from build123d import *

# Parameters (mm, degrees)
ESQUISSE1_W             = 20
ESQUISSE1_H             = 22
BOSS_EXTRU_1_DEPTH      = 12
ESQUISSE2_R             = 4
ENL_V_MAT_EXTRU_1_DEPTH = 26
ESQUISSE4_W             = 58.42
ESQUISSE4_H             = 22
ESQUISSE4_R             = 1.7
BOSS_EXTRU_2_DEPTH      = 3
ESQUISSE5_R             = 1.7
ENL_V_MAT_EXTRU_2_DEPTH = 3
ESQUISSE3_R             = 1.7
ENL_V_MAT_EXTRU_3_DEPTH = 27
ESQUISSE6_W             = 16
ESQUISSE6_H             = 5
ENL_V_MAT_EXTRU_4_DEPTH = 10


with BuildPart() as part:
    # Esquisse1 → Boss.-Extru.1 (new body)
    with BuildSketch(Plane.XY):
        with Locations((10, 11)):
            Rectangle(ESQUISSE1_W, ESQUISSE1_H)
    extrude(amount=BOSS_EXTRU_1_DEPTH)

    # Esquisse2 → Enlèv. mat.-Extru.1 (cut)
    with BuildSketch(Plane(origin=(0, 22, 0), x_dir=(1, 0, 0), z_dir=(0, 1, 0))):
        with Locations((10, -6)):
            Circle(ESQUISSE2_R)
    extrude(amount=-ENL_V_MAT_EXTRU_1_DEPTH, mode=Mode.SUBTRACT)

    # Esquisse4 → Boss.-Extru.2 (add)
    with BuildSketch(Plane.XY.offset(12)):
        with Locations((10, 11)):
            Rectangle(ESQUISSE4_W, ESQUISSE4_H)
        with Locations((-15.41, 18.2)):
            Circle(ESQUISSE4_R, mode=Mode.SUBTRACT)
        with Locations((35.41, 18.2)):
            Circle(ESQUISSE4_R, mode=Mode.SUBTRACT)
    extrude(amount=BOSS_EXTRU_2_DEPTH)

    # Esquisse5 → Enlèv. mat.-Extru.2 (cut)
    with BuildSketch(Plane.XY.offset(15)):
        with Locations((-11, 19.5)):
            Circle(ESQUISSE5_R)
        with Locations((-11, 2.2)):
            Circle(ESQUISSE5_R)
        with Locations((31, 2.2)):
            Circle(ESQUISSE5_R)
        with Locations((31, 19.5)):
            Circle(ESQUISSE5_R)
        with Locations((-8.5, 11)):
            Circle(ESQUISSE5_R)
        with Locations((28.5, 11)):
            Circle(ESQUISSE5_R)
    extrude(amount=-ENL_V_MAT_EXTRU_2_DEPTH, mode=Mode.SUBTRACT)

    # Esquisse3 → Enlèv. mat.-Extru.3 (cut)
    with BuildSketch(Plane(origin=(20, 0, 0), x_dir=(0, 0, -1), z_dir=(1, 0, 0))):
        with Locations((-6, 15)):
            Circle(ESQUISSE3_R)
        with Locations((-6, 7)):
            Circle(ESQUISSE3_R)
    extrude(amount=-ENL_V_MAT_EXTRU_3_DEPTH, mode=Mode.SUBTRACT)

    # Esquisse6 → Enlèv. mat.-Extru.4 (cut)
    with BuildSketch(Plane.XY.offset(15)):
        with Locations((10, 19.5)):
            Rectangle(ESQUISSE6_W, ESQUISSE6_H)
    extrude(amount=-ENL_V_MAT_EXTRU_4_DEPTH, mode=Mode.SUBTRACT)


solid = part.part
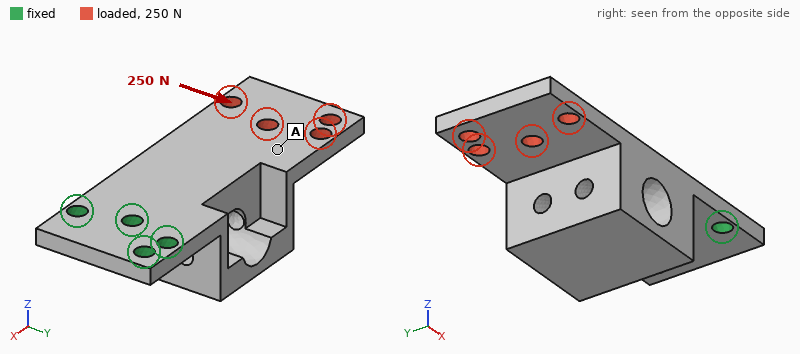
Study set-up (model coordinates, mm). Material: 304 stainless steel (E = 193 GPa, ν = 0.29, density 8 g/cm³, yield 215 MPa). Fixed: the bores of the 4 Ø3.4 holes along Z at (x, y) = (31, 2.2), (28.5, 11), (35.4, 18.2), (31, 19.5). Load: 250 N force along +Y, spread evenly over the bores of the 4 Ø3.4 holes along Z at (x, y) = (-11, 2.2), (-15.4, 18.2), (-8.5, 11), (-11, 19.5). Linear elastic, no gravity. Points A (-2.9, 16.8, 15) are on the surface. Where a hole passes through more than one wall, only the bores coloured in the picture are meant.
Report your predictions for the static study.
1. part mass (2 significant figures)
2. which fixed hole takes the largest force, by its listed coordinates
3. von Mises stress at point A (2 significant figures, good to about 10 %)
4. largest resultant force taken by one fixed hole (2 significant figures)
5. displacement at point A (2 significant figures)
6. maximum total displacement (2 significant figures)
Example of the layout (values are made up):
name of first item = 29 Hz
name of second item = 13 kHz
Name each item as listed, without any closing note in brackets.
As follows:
part mass = 56 g
which fixed hole takes the largest force, by its listed coordinates = (31, 2.2)
von Mises stress at point A = 7.5 MPa
largest resultant force taken by one fixed hole = 590 N
displacement at point A = 13 µm
maximum total displacement = 23 µm
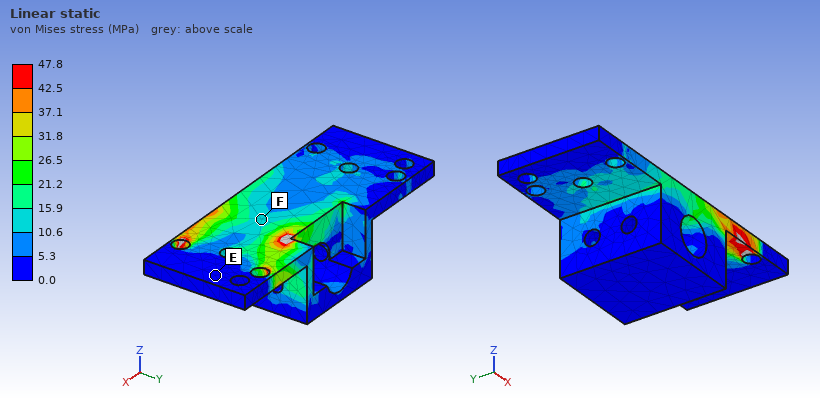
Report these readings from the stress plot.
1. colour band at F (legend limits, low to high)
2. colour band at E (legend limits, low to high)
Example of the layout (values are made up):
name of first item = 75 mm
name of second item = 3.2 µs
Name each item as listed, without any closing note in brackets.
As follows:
colour band at F = 10.6 to 15.9 MPa
colour band at E = 0.0 to 5.3 MPa
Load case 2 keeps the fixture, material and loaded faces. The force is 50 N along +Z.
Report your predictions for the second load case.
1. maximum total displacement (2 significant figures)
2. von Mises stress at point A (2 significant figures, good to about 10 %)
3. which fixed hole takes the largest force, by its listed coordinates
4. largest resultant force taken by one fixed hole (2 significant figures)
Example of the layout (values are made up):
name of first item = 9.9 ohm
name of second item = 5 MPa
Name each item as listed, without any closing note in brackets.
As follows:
maximum total displacement = 90 µm
von Mises stress at point A = 13 MPa
which fixed hole takes the largest force, by its listed coordinates = (28.5, 11)
largest resultant force taken by one fixed hole = 130 N
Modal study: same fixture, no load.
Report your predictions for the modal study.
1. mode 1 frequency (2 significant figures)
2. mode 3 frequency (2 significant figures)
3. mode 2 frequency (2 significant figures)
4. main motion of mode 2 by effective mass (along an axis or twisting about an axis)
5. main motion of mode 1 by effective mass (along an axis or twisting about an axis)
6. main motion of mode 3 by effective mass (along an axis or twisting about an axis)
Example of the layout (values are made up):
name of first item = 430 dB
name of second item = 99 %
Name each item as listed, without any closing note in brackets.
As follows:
mode 1 frequency = 1100 Hz
mode 3 frequency = 5500 Hz
mode 2 frequency = 4500 Hz
main motion of mode 2 by effective mass = along Y
main motion of mode 1 by effective mass = along Z
main motion of mode 3 by effective mass = along Y
